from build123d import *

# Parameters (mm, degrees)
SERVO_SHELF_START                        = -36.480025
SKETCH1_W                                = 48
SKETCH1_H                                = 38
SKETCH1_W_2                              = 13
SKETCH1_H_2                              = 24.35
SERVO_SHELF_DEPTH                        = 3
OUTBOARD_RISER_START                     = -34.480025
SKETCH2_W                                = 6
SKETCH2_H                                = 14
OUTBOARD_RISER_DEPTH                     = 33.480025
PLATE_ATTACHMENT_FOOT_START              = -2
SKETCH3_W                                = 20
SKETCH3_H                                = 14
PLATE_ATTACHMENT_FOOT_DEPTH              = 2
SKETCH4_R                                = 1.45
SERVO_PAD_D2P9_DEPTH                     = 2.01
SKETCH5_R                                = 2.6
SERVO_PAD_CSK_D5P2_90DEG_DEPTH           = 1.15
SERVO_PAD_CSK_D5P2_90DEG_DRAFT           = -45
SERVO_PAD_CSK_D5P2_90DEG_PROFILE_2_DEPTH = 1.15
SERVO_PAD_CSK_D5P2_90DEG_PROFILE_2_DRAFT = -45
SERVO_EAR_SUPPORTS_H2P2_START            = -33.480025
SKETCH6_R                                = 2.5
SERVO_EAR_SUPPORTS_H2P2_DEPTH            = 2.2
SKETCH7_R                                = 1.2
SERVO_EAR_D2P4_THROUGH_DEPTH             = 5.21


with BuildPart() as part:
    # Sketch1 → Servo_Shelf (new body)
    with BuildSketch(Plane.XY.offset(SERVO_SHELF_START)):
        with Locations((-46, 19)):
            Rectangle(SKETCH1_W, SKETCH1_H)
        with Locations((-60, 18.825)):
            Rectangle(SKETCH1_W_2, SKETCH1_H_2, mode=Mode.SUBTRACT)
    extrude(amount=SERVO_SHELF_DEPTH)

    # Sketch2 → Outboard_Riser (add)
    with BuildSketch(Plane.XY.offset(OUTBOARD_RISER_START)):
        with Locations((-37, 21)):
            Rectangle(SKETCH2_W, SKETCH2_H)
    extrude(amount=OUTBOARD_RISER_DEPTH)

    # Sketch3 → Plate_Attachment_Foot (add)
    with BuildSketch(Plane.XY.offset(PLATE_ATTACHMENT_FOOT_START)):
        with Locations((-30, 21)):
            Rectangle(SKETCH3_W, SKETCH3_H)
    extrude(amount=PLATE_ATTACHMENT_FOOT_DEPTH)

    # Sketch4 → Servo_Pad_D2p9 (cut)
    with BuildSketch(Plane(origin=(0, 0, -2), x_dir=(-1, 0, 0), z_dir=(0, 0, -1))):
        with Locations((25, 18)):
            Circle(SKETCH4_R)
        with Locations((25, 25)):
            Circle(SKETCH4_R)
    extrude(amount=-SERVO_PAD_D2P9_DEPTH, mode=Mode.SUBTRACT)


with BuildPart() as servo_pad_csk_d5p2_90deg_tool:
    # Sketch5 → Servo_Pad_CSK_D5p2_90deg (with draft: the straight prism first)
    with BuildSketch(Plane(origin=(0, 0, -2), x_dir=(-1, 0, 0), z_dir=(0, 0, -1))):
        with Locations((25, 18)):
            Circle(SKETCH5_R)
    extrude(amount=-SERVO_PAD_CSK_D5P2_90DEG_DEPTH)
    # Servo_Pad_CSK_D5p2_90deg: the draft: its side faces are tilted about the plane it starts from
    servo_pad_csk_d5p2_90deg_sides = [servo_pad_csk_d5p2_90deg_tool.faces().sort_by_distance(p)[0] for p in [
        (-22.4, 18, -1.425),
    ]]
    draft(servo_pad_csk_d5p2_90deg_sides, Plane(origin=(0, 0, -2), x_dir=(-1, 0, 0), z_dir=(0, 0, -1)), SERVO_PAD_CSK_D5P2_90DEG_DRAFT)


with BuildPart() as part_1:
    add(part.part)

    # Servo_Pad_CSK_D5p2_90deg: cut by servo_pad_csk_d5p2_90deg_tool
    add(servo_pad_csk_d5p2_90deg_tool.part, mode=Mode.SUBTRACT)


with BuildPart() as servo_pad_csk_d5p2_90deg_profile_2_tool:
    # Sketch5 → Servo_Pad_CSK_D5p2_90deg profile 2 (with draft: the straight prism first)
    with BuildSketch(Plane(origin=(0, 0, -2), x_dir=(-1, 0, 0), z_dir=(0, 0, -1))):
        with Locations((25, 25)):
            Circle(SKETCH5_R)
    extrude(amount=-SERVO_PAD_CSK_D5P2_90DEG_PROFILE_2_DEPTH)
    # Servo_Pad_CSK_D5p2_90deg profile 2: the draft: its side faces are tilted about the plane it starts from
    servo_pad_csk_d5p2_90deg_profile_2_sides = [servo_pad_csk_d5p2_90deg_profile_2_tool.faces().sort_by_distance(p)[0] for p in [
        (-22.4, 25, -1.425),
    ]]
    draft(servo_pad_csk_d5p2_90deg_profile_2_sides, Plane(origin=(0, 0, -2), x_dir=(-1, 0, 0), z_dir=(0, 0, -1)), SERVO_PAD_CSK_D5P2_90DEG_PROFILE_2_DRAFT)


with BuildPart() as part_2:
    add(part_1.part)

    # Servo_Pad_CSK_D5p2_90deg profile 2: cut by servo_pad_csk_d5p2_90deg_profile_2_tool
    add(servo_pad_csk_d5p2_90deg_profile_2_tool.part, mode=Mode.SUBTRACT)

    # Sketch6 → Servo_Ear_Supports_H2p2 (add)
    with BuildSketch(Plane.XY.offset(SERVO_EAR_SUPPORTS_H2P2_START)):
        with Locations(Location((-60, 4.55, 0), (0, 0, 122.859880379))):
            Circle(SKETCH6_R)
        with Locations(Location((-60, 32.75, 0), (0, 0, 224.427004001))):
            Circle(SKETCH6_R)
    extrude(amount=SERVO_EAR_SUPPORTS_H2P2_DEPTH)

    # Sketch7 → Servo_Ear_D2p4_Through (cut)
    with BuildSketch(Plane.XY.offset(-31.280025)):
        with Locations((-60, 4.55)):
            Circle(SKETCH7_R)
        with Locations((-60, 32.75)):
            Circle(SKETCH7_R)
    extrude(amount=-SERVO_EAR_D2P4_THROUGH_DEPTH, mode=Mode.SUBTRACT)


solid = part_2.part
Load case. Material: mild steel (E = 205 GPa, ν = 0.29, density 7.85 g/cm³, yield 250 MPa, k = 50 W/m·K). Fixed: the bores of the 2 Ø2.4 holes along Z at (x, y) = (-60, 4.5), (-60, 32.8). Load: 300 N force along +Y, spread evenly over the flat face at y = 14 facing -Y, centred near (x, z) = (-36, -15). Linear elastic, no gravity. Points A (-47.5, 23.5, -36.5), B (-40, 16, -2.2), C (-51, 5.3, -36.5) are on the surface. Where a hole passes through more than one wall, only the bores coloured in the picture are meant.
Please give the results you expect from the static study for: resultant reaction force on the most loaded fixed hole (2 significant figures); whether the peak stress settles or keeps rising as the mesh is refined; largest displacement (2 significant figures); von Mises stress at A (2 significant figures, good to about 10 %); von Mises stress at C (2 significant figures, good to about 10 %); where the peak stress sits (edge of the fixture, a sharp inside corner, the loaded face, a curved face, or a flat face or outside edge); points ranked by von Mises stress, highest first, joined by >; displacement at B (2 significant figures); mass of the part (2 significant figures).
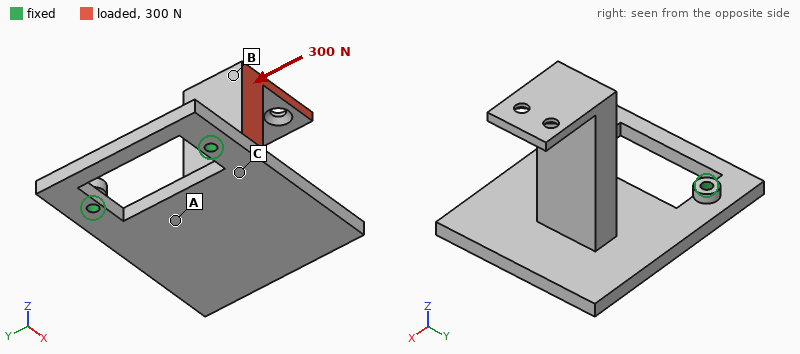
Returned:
310 N
keeps rising
0.12 mm
65 MPa
36 MPa
edge of the fixture
A > C > B
0.11 mm
61 g
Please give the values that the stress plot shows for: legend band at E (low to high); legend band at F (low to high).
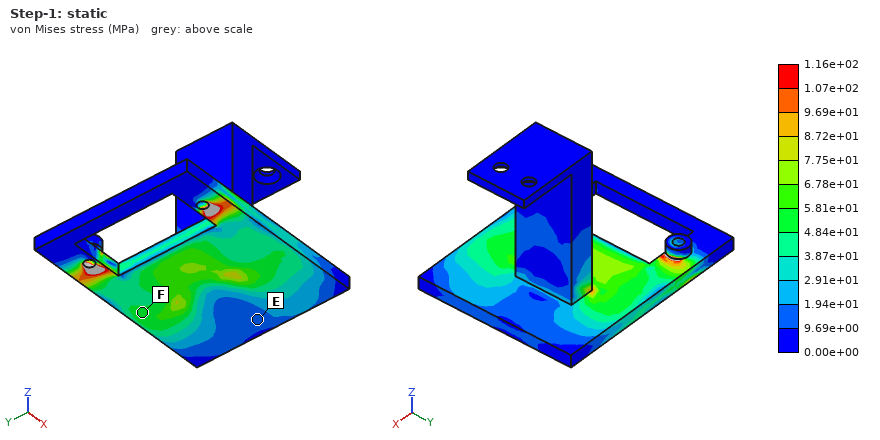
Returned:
9.69e+00 to 1.94e+01 MPa
4.84e+01 to 5.81e+01 MPa
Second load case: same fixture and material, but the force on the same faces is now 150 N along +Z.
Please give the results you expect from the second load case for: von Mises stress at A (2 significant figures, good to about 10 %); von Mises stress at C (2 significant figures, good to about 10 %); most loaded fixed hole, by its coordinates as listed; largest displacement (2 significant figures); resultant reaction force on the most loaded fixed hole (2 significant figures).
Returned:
22 MPa
87 MPa
(-60, 4.5)
0.26 mm
98 N
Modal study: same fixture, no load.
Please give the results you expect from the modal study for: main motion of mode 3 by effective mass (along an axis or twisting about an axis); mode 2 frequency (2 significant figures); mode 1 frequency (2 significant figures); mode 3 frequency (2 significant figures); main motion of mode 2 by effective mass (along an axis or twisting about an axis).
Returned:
along Z
1800 Hz
650 Hz
2700 Hz
along Y
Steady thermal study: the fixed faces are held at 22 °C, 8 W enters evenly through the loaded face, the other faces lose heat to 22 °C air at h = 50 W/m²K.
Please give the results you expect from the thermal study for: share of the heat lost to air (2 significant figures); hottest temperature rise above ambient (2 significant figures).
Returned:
68 %
46 K
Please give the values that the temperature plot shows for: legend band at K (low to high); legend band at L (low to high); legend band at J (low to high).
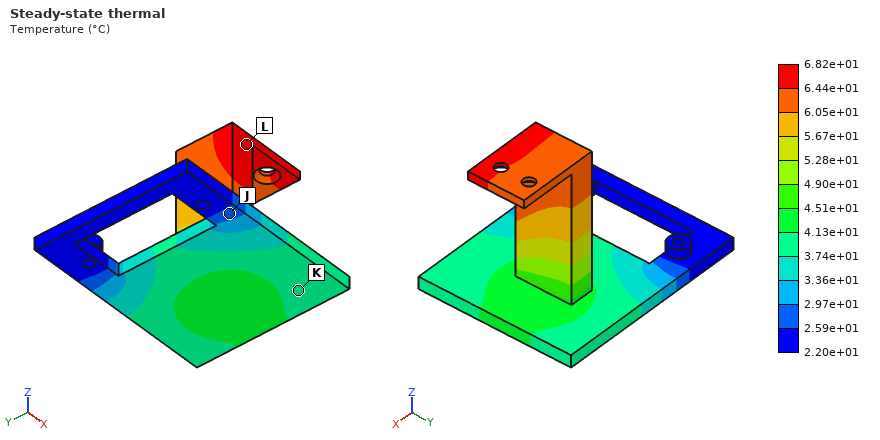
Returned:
3.74e+01 to 4.13e+01 °C
6.44e+01 to 6.82e+01 °C
2.59e+01 to 2.97e+01 °C
